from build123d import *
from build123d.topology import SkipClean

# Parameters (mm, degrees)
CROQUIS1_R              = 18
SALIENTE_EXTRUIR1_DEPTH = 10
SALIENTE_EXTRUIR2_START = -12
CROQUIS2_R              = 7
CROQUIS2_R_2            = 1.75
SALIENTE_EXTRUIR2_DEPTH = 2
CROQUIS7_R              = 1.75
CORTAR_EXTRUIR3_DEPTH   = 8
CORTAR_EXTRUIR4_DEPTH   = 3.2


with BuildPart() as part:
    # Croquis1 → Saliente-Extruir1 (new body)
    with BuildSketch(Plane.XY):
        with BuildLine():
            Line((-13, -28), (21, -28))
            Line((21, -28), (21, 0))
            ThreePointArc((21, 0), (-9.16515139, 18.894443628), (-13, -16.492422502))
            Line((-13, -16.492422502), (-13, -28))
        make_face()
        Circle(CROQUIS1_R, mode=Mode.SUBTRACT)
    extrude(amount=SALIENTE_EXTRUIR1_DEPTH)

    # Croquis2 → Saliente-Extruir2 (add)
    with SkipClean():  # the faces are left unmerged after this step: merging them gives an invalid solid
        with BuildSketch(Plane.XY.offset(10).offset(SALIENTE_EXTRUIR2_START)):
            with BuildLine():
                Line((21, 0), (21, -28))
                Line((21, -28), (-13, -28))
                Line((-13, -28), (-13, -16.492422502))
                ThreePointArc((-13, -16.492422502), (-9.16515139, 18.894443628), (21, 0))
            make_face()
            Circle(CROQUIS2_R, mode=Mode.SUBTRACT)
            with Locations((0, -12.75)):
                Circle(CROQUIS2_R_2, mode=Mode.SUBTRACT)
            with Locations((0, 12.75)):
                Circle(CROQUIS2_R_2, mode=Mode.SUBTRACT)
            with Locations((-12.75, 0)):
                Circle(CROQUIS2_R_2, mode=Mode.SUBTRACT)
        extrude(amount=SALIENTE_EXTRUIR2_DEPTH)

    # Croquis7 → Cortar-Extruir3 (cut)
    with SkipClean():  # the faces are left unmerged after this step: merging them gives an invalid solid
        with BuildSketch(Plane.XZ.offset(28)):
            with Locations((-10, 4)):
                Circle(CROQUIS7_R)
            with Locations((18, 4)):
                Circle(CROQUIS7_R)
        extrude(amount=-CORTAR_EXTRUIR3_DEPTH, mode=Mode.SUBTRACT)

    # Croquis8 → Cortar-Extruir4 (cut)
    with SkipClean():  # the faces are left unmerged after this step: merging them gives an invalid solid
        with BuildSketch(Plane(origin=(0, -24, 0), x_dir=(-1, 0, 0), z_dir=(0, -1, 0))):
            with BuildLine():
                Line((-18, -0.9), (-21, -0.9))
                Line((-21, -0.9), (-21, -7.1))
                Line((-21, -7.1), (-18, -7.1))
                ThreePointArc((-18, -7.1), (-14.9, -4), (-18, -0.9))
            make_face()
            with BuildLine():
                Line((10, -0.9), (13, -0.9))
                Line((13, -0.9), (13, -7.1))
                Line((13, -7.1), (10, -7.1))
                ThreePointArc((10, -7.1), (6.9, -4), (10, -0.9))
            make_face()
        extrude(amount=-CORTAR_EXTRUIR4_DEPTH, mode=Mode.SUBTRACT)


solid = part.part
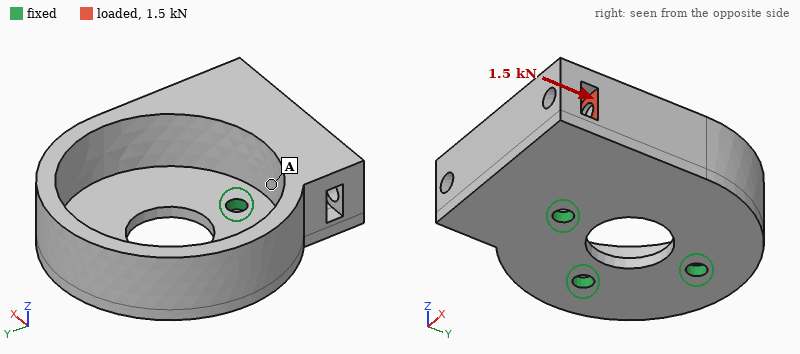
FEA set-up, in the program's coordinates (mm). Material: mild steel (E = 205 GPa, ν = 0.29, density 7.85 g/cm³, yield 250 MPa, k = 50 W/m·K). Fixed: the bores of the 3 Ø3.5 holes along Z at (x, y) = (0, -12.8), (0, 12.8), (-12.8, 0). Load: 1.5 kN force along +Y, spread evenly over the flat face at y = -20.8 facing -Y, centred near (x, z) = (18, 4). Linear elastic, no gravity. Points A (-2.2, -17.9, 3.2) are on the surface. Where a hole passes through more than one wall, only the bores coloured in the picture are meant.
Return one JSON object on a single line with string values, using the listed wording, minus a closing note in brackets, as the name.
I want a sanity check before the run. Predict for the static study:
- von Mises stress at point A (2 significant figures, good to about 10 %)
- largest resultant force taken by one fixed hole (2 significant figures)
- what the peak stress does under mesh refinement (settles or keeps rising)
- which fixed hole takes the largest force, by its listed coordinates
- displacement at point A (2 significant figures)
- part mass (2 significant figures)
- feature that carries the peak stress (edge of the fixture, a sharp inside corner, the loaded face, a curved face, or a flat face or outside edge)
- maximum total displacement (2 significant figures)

{"von Mises stress at point A": "17 MPa", "largest resultant force taken by one fixed hole": "1.3 kN", "what the peak stress does under mesh refinement": "keeps rising", "which fixed hole takes the largest force, by its listed coordinates": "(0, -12.8)", "displacement at point A": "5.2 µm", "part mass": "78 g", "feature that carries the peak stress": "edge of the fixture", "maximum total displacement": "24 µm"}
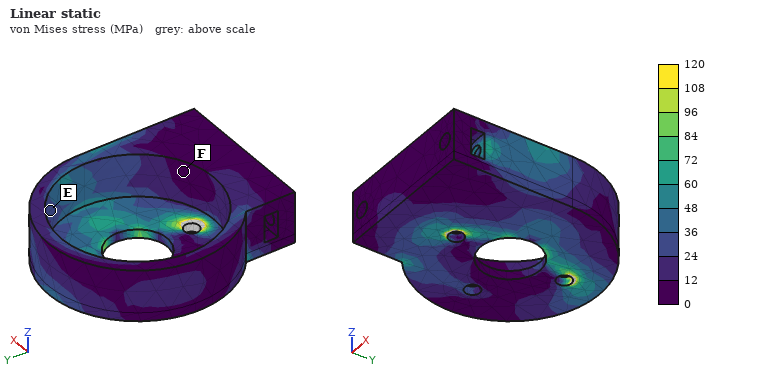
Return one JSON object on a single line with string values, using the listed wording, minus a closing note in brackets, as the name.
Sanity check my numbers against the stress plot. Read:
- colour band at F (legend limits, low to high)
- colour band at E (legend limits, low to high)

{"colour band at F": "0 to 12 MPa", "colour band at E": "24 to 36 MPa"}
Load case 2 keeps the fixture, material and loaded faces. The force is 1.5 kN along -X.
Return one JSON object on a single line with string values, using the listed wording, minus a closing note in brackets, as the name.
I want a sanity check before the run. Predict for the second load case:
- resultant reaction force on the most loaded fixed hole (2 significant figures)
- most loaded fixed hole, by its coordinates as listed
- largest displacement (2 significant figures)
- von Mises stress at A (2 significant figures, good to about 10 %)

{"resultant reaction force on the most loaded fixed hole": "1.7 kN", "most loaded fixed hole, by its coordinates as listed": "(0, -12.8)", "largest displacement": "23 µm", "von Mises stress at A": "30 MPa"}
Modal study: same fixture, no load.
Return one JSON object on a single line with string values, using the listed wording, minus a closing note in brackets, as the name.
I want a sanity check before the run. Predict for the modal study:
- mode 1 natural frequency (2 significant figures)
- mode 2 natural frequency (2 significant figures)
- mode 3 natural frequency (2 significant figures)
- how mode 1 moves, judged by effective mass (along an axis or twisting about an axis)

{"mode 1 natural frequency": "4000 Hz", "mode 2 natural frequency": "5600 Hz", "mode 3 natural frequency": "9600 Hz", "how mode 1 moves, judged by effective mass": "along Z"}
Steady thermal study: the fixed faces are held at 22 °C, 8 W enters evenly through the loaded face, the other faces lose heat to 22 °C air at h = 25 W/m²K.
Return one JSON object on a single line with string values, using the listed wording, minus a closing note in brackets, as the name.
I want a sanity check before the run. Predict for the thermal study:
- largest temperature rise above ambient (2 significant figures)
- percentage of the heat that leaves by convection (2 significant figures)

{"largest temperature rise above ambient": "40 K", "percentage of the heat that leaves by convection": "21 %"}
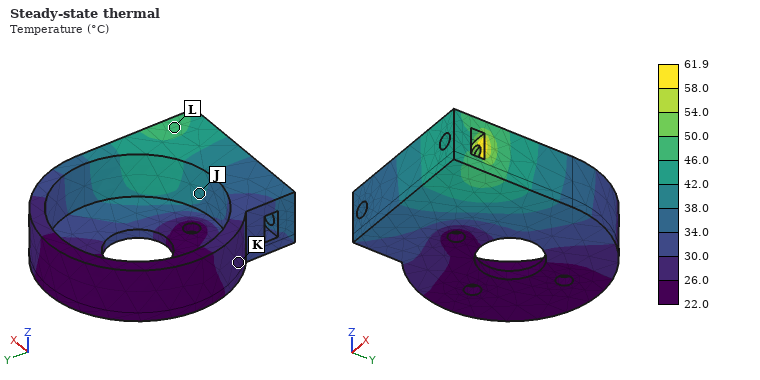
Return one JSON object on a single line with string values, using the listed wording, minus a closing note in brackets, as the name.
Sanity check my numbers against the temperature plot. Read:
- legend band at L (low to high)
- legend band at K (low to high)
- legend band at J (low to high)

{"legend band at L": "46.0 to 50.0 °C", "legend band at K": "26.0 to 30.0 °C", "legend band at J": "38.0 to 42.0 °C"}
